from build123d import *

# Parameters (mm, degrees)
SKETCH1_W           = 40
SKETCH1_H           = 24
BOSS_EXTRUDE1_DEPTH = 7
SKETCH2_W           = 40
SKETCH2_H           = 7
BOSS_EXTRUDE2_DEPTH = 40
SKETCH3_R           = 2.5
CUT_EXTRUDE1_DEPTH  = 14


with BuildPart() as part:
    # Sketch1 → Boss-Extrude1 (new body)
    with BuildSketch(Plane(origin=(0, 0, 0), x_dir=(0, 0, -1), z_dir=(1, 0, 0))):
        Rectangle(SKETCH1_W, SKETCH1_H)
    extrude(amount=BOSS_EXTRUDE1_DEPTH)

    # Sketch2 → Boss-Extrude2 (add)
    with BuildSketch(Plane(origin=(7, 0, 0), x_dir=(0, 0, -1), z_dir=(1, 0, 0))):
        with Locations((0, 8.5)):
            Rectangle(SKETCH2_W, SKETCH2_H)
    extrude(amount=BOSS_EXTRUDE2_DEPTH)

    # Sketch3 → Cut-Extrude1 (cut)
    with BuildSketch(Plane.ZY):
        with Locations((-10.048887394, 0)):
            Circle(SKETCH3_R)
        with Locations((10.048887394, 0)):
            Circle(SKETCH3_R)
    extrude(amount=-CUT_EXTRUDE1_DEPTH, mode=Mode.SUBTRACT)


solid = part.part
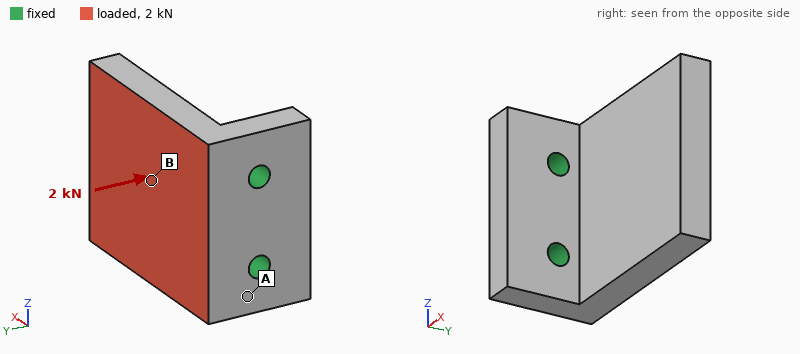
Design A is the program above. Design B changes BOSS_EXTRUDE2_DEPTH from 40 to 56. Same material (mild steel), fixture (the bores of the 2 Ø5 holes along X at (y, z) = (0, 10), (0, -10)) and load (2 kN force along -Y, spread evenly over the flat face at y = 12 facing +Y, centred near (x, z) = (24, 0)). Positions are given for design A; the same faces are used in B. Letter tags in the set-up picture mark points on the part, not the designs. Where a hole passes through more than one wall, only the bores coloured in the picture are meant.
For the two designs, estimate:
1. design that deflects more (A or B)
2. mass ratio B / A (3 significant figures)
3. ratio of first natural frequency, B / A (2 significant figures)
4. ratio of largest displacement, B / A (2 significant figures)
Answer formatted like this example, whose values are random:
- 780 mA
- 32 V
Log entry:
- B
- 1.25
- 0.57
- 2.3
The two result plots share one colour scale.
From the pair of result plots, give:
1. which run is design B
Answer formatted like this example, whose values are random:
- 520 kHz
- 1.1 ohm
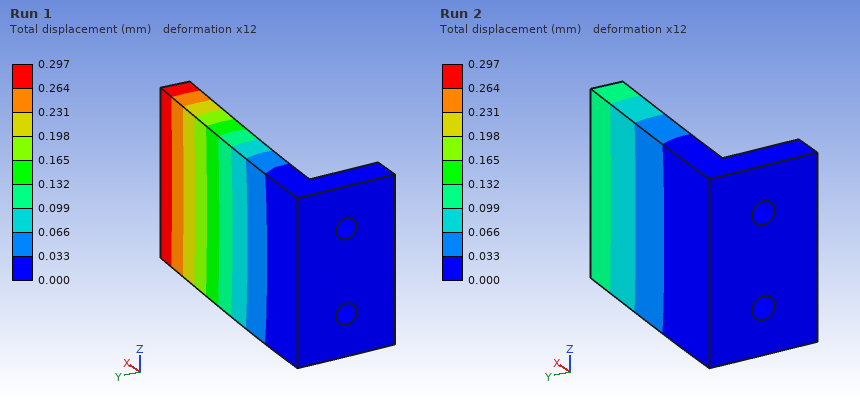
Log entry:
- Run 1
